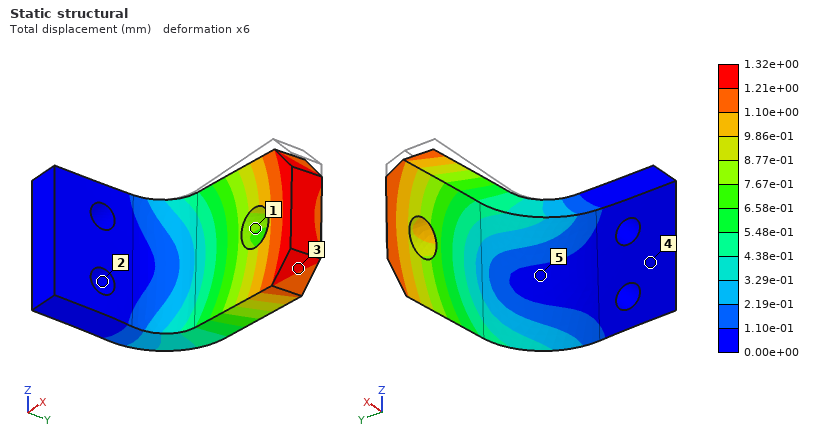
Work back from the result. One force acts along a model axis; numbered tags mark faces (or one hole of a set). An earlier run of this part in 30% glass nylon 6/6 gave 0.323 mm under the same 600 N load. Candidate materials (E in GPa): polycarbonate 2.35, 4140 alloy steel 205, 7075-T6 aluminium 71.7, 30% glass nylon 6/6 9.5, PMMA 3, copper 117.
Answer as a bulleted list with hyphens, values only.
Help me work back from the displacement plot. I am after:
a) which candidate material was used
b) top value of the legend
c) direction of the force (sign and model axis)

- polycarbonate
- 1.32e+00 mm
- -Z
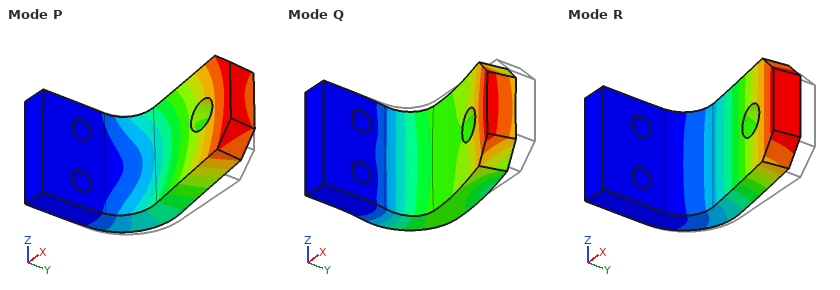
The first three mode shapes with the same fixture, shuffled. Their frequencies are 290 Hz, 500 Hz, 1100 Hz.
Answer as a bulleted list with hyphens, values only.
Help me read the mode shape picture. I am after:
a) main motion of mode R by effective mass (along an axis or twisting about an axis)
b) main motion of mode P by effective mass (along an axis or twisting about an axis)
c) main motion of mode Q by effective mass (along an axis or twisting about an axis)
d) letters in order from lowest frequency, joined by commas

- along Y
- along Z
- along X
- R, P, Q
